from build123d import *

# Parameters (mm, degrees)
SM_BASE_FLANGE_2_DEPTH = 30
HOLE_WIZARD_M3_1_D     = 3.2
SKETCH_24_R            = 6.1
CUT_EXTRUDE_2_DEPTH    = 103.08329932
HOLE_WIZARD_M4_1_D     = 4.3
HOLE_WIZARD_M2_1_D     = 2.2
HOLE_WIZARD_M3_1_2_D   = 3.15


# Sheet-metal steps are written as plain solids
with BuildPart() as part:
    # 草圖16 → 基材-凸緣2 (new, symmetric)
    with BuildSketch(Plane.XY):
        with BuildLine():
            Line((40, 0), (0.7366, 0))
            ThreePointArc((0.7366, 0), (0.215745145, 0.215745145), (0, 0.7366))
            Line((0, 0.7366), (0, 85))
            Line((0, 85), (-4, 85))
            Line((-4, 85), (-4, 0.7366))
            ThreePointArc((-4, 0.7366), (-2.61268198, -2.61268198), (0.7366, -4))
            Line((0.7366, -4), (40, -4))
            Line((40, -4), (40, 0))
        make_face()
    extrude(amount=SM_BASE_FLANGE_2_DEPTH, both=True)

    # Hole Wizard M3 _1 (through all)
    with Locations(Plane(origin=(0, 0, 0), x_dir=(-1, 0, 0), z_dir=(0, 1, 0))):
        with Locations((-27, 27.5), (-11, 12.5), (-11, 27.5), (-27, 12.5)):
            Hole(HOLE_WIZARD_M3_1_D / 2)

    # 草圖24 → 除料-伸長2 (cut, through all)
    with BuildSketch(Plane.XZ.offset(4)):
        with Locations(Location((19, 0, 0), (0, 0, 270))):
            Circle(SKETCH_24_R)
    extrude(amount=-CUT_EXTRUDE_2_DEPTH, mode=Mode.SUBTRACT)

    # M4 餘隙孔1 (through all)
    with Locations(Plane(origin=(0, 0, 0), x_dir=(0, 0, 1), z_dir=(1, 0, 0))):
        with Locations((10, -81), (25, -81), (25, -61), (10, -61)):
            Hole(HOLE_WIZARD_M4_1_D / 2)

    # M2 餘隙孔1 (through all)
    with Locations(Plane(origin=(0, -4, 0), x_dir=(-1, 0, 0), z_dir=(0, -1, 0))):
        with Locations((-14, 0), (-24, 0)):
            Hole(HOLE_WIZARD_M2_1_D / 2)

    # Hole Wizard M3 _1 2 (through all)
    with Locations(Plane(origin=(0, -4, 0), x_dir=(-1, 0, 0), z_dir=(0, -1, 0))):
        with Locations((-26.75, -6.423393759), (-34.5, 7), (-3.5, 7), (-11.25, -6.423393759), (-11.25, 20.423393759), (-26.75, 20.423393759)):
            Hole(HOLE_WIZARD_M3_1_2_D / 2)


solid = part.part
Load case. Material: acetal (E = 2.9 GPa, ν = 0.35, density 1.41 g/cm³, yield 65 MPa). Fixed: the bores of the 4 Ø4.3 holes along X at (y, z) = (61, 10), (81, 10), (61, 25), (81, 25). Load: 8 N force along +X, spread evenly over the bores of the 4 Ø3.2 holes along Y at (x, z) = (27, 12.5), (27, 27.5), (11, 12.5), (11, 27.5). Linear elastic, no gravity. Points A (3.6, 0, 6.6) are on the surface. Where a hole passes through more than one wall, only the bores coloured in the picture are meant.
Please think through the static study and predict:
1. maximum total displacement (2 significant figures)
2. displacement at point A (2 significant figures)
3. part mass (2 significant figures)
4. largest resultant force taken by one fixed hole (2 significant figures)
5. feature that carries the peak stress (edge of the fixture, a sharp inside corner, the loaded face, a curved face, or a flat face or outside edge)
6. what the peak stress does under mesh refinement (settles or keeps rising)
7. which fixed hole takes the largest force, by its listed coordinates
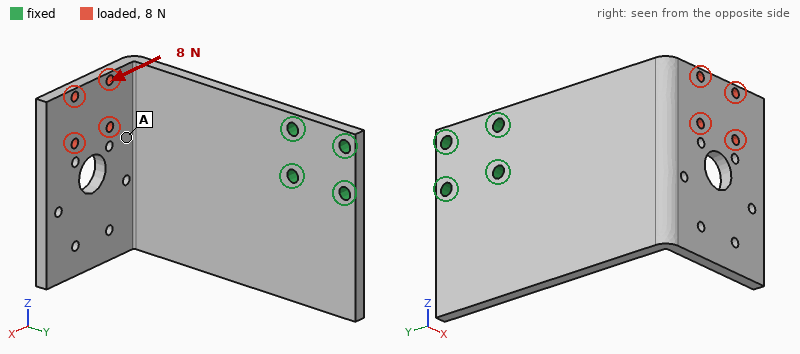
1.2 mm
0.76 mm
42 g
13 N
edge of the fixture
keeps rising
(61, 10)
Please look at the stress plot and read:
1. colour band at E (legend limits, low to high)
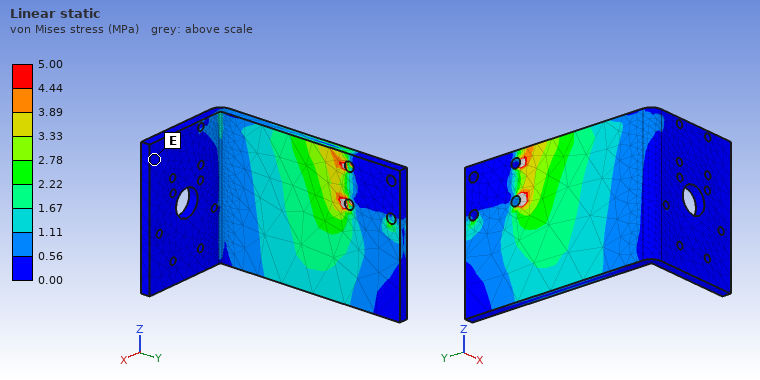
0.00 to 0.56 MPa
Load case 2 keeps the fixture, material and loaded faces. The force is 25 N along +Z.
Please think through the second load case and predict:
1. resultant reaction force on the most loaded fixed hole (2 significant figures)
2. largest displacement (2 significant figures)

57 N
1.3 mm
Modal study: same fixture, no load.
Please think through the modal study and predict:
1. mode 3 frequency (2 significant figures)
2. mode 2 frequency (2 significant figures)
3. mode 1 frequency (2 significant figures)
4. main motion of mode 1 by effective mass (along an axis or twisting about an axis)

350 Hz
200 Hz
110 Hz
along X
